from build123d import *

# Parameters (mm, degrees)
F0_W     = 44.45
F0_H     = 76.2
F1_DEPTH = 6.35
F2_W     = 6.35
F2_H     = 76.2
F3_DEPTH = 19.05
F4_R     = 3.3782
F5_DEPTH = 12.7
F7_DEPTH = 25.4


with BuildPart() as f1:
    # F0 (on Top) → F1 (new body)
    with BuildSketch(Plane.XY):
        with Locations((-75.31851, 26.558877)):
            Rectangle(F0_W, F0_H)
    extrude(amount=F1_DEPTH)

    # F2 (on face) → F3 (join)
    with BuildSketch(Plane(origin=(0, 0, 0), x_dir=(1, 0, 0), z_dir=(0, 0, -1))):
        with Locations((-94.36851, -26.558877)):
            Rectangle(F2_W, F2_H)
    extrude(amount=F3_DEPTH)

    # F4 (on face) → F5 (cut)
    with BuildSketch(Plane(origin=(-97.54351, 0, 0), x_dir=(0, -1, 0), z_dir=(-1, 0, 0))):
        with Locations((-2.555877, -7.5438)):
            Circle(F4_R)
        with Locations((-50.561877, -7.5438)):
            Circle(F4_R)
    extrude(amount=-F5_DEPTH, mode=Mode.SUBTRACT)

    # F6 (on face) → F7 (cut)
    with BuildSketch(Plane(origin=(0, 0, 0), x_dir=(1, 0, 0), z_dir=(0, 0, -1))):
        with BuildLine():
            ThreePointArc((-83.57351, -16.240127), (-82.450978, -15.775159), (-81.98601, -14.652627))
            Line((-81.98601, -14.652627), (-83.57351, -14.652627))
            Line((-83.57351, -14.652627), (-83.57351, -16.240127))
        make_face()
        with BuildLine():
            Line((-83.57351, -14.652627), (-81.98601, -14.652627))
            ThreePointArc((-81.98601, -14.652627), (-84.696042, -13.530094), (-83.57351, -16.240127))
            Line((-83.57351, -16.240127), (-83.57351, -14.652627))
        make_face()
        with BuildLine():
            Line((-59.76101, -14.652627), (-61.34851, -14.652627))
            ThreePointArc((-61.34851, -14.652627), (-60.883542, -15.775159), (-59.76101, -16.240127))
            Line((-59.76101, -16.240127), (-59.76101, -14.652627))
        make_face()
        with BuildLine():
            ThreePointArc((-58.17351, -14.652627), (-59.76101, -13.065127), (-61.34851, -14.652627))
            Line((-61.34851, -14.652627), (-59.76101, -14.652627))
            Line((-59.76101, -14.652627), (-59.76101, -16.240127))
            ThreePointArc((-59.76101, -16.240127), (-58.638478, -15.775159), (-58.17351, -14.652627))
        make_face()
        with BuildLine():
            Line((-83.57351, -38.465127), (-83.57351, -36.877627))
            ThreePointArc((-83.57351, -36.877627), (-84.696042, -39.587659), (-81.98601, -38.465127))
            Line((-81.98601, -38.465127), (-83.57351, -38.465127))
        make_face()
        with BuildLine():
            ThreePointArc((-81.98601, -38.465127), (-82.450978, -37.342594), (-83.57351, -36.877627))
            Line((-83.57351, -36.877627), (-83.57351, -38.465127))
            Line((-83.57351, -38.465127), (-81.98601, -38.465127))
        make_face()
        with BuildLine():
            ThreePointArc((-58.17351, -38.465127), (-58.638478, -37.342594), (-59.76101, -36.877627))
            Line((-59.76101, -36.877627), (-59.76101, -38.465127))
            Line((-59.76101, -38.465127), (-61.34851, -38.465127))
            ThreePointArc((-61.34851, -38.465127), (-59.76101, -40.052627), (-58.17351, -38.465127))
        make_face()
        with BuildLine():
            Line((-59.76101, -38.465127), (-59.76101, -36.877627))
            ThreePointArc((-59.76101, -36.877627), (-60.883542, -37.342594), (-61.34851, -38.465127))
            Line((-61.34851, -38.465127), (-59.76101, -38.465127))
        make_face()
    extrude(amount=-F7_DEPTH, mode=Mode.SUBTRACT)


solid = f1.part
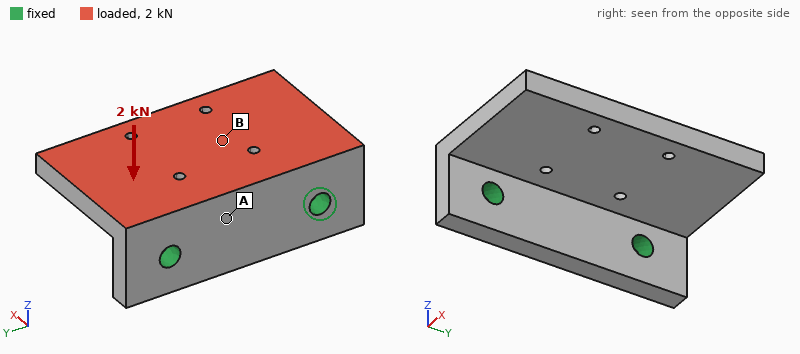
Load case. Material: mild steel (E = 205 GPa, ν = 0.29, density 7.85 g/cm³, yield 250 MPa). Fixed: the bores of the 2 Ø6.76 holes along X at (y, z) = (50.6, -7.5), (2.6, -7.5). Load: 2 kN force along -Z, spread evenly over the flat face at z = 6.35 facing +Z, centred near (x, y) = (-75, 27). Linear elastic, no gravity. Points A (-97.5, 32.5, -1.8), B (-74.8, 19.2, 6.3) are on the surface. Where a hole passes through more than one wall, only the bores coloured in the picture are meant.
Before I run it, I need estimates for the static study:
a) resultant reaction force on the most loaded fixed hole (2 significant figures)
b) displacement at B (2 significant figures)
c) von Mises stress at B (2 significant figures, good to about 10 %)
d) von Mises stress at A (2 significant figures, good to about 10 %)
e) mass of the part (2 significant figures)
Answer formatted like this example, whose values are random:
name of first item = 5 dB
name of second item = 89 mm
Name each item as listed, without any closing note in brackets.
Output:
resultant reaction force on the most loaded fixed hole = 1.0 kN
displacement at B = 41 µm
von Mises stress at B = 18 MPa
von Mises stress at A = 43 MPa
mass of the part = 240 g
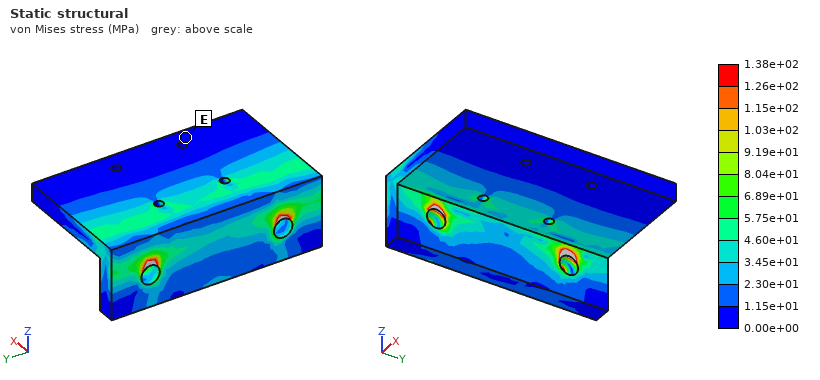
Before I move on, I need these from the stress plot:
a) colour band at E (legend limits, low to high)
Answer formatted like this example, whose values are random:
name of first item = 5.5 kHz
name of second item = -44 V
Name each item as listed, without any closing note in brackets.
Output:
colour band at E = 0.00e+00 to 1.15e+01 MPa
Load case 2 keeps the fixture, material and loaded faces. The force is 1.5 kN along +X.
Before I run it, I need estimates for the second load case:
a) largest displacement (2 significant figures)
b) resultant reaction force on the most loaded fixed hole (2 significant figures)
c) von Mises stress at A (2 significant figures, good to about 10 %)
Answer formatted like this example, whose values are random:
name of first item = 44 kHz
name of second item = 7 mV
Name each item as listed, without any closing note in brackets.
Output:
largest displacement = 26 µm
resultant reaction force on the most loaded fixed hole = 750 N
von Mises stress at A = 11 MPa
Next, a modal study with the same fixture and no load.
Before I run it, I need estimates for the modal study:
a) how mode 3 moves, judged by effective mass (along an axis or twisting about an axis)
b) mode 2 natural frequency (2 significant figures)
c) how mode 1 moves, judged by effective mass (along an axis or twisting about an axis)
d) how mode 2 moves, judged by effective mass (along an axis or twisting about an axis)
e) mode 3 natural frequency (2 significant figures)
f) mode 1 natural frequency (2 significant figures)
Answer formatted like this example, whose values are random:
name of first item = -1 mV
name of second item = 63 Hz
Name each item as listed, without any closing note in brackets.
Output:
how mode 3 moves, judged by effective mass = along Y
mode 2 natural frequency = 4100 Hz
how mode 1 moves, judged by effective mass = along Z
how mode 2 moves, judged by effective mass = twisting about X
mode 3 natural frequency = 8000 Hz
mode 1 natural frequency = 2200 Hz
